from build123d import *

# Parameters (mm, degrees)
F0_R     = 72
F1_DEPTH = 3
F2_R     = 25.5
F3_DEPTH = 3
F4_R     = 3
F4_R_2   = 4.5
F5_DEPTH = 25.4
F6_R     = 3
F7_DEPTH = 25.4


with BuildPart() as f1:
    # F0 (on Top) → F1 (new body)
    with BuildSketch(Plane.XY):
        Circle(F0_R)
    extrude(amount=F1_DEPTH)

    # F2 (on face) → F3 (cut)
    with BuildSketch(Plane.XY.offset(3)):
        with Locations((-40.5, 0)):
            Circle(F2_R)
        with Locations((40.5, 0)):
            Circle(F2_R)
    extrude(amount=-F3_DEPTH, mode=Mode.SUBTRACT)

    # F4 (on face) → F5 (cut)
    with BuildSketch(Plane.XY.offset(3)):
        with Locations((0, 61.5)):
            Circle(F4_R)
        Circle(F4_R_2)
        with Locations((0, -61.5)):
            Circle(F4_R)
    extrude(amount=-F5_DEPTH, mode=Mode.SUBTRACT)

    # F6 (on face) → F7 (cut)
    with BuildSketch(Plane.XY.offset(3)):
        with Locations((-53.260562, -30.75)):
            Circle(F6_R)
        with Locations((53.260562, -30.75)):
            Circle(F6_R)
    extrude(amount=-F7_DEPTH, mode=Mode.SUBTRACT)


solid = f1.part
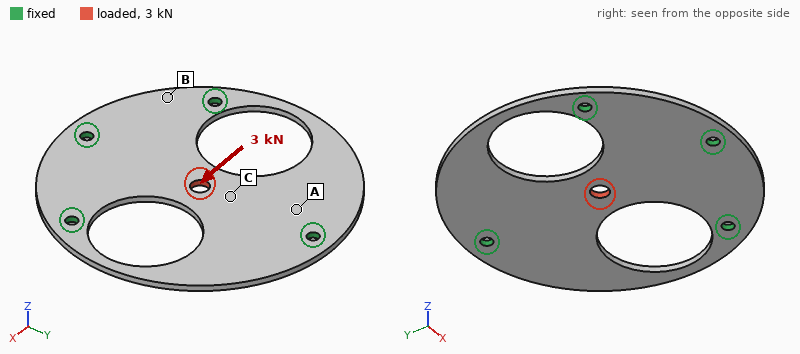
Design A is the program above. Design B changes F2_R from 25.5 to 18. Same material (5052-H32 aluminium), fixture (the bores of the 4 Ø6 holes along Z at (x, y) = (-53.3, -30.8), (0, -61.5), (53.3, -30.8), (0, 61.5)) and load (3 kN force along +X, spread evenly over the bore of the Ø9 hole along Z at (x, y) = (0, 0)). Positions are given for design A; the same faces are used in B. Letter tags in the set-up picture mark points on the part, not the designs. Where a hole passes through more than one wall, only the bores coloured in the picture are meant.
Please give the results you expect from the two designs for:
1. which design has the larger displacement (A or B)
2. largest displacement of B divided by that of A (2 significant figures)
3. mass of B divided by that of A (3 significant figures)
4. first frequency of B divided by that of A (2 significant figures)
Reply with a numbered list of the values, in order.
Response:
1. A
2. 0.54
3. 1.17
4. 1.1
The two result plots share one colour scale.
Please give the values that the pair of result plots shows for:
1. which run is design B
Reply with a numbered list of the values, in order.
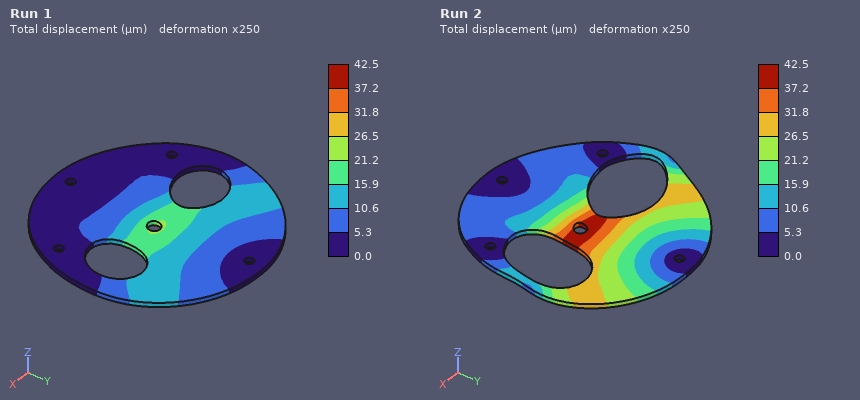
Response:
1. Run 1
